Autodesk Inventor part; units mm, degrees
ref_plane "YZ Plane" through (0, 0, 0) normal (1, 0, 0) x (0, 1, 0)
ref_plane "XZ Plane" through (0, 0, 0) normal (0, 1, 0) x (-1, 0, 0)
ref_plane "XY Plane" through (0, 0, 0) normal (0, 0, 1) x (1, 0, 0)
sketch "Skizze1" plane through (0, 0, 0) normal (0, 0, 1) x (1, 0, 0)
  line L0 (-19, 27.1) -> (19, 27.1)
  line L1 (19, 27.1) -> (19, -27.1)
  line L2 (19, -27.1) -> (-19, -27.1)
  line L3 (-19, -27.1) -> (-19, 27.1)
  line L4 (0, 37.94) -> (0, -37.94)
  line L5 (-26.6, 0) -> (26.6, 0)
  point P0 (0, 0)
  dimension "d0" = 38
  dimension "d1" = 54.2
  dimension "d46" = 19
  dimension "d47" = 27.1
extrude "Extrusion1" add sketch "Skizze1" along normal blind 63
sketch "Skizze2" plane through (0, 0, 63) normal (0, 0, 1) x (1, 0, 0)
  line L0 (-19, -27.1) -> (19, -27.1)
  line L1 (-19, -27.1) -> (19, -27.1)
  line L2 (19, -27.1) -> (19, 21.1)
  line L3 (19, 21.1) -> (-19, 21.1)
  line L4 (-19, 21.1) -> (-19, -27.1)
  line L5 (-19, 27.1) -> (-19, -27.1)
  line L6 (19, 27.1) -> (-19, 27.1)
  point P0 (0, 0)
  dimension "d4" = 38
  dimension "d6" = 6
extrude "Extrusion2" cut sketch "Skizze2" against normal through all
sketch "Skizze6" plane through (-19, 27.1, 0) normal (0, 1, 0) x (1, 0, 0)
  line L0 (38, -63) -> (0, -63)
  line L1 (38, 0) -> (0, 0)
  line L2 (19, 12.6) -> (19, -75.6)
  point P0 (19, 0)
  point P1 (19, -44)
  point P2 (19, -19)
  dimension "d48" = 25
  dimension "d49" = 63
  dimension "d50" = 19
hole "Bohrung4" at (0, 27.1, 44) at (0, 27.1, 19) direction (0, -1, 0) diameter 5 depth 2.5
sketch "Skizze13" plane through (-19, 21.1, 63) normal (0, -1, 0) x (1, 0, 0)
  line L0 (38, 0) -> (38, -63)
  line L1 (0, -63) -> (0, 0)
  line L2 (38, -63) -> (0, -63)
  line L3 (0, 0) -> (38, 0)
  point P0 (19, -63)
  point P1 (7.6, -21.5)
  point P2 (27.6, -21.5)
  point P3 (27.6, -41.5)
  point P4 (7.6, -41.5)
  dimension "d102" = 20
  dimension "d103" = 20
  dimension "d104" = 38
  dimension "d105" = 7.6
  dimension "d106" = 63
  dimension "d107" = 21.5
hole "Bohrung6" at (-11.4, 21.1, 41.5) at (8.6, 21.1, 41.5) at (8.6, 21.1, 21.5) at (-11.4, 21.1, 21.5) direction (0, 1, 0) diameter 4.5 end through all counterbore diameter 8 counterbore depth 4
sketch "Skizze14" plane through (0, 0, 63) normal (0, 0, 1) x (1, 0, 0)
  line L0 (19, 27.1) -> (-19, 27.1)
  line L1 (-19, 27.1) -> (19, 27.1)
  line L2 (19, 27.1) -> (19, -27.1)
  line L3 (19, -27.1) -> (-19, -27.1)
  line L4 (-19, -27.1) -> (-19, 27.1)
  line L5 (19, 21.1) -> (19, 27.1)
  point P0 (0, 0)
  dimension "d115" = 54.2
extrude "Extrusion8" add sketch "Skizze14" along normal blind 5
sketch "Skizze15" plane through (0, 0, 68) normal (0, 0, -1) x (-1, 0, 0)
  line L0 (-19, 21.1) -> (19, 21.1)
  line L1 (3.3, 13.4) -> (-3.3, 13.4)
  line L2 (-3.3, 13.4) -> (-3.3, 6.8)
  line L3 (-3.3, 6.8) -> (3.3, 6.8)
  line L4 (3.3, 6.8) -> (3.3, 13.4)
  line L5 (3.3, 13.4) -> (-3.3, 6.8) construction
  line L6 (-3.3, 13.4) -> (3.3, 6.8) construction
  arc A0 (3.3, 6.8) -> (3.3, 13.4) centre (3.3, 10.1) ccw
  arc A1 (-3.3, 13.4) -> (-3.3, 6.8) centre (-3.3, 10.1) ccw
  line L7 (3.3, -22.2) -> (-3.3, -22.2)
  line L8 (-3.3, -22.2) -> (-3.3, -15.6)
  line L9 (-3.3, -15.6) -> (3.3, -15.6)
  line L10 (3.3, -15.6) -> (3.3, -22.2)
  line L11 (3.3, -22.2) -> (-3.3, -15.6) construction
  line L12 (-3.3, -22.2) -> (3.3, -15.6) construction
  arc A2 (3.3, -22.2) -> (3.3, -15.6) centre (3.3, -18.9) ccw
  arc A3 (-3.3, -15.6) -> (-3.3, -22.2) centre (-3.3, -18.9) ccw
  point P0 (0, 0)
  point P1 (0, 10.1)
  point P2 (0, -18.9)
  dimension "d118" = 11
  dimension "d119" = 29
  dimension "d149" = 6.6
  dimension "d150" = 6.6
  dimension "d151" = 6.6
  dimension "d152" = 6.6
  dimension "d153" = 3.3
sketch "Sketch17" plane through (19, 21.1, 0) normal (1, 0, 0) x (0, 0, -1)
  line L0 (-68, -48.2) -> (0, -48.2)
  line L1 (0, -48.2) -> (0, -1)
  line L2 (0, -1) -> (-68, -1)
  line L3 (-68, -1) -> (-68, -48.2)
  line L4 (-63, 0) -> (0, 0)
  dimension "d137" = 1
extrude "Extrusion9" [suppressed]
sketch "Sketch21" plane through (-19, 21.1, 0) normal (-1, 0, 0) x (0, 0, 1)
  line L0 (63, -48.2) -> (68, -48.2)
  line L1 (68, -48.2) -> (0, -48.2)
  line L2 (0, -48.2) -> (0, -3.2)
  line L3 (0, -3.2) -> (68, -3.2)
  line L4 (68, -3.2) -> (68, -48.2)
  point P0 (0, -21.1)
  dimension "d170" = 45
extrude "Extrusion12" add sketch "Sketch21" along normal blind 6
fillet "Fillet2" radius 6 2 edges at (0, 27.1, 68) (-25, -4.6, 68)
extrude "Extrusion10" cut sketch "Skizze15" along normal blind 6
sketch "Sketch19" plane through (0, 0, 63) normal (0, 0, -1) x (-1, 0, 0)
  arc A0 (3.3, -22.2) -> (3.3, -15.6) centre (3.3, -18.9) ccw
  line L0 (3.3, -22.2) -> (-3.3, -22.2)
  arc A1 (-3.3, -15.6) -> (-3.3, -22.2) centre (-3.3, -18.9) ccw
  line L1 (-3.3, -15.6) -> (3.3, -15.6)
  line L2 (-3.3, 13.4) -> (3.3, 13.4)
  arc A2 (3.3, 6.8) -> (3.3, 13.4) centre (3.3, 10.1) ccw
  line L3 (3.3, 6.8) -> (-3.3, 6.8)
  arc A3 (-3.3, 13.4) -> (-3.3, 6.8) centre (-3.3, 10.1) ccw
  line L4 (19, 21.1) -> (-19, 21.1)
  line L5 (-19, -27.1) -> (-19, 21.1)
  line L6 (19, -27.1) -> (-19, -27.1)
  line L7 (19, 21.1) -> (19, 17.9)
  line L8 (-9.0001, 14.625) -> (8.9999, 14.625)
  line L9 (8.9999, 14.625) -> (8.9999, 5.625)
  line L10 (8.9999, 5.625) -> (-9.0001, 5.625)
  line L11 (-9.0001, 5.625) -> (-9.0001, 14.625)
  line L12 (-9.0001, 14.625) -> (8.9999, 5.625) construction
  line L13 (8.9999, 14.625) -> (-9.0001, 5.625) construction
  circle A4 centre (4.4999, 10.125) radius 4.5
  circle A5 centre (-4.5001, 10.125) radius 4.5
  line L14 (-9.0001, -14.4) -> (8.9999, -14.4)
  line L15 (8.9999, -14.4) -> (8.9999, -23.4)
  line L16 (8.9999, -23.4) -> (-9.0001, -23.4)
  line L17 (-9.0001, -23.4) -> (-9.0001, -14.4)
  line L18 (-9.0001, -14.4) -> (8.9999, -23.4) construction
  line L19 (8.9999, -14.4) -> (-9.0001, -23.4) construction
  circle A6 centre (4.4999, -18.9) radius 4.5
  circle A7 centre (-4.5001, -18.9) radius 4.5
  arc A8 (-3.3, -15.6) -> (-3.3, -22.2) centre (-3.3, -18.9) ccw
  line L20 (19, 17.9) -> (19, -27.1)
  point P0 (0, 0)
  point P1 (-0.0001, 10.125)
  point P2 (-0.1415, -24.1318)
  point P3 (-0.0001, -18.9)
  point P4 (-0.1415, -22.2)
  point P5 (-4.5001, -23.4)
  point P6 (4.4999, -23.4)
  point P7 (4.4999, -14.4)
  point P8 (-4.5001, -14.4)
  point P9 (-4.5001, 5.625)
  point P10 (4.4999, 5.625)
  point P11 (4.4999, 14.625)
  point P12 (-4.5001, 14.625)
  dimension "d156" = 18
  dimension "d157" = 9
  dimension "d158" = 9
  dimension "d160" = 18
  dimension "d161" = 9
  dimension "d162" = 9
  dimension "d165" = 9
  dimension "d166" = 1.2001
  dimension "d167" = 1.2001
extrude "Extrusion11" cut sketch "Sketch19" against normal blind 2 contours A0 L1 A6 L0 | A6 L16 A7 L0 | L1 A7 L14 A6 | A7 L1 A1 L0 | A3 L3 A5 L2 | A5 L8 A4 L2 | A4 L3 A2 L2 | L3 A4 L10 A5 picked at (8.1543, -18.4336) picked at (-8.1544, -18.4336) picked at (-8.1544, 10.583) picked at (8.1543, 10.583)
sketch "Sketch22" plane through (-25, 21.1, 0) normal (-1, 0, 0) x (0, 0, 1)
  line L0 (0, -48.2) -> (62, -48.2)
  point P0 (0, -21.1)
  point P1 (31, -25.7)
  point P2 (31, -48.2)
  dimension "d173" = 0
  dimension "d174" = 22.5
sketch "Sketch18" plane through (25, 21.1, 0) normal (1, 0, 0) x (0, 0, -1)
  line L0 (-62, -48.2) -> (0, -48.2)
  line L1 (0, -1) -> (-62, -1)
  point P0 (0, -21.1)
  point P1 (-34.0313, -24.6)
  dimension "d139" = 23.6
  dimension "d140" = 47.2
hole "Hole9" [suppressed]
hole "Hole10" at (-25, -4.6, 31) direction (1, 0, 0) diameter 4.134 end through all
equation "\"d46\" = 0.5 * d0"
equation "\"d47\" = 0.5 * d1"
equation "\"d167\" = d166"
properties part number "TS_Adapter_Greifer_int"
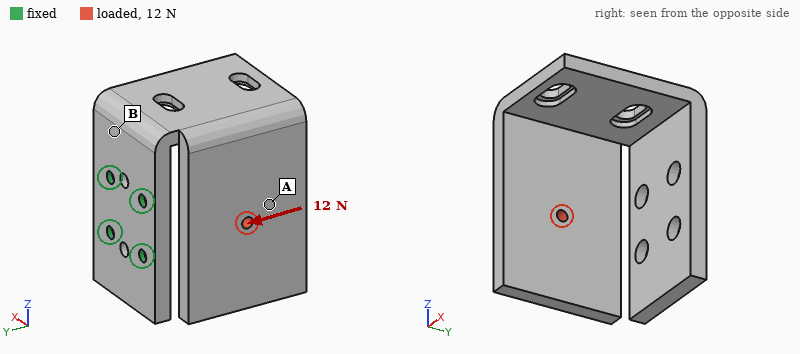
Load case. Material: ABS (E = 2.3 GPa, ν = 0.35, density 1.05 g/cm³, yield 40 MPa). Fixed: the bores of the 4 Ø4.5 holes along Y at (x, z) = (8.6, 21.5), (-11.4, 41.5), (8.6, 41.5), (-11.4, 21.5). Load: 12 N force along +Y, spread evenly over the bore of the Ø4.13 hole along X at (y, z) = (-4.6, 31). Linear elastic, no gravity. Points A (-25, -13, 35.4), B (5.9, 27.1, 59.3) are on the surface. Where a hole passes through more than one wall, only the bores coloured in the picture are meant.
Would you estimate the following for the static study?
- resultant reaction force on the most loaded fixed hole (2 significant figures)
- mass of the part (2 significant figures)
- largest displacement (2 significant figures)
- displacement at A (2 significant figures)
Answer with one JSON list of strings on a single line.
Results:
["16 N", "42 g", "1.2 mm", "0.63 mm"]
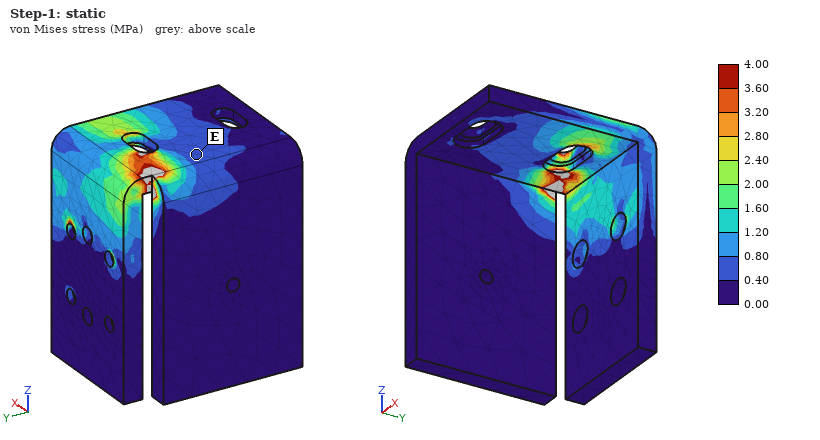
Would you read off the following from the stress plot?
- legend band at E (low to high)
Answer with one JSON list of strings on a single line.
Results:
["0.40 to 0.80 MPa"]
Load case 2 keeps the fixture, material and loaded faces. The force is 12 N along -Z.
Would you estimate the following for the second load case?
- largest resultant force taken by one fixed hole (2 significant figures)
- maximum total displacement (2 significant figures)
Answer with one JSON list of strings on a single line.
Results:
["19 N", "1.1 mm"]
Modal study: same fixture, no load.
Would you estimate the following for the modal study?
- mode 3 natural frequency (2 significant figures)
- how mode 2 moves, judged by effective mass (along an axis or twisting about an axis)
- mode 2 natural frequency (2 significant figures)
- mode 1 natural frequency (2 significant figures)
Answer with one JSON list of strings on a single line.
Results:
["360 Hz", "along X", "160 Hz", "120 Hz"]
